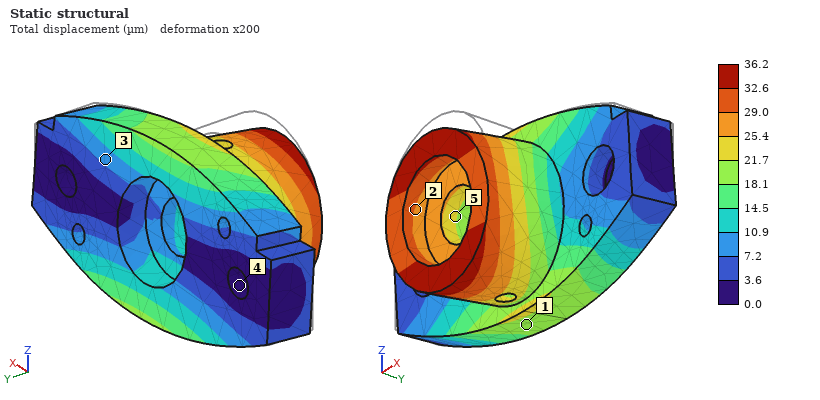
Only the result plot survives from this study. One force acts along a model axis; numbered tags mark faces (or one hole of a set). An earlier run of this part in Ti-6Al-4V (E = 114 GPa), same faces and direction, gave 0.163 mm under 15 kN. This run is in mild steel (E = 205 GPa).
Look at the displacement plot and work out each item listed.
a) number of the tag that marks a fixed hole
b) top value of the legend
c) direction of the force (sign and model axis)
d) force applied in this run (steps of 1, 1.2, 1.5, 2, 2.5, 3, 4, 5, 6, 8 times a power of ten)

4
36.2 µm
-Z
6 kN
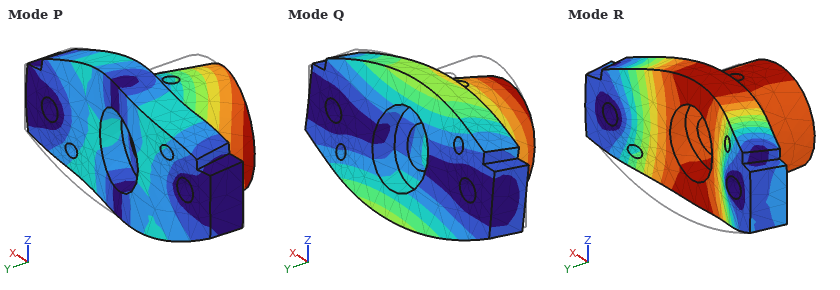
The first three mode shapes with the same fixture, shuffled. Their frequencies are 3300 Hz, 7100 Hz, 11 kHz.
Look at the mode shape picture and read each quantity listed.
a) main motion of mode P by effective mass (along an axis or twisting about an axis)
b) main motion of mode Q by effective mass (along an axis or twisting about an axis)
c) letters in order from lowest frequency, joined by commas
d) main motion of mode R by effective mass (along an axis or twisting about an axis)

along X
along Z
Q, R, P
along Y
